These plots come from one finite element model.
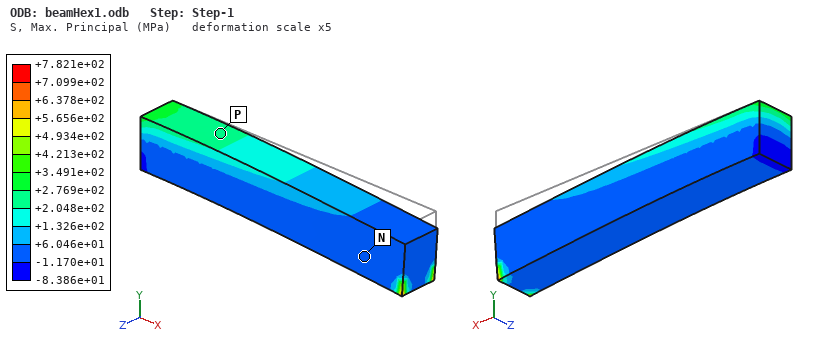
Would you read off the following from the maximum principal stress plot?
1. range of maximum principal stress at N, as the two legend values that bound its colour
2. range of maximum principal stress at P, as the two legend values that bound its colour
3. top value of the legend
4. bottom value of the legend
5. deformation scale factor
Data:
-1.170e+01 to +6.046e+01 MPa
+2.048e+02 to +2.769e+02 MPa
+7.821e+02 MPa
-8.386e+01 MPa
5
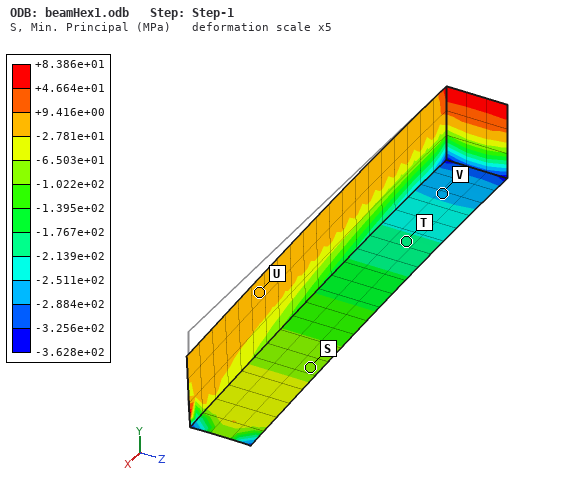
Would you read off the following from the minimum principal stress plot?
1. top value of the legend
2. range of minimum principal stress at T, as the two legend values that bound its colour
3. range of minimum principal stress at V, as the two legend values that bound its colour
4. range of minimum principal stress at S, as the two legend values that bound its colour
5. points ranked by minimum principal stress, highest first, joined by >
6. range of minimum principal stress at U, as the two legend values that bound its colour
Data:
+8.386e+01 MPa
-2.139e+02 to -1.767e+02 MPa
-2.884e+02 to -2.511e+02 MPa
-1.022e+02 to -6.503e+01 MPa
U > S > T > V
-2.781e+01 to +9.416e+00 MPa
